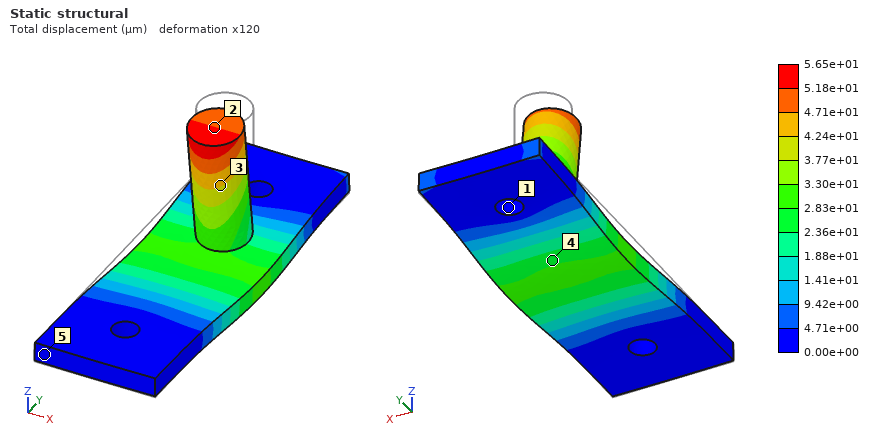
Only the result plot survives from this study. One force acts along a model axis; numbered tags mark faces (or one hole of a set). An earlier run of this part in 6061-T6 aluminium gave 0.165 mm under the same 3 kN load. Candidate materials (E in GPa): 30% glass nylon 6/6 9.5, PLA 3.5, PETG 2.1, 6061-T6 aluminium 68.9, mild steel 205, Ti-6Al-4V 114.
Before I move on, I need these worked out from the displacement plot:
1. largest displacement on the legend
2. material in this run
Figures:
5.65e+01 µm
mild steel
